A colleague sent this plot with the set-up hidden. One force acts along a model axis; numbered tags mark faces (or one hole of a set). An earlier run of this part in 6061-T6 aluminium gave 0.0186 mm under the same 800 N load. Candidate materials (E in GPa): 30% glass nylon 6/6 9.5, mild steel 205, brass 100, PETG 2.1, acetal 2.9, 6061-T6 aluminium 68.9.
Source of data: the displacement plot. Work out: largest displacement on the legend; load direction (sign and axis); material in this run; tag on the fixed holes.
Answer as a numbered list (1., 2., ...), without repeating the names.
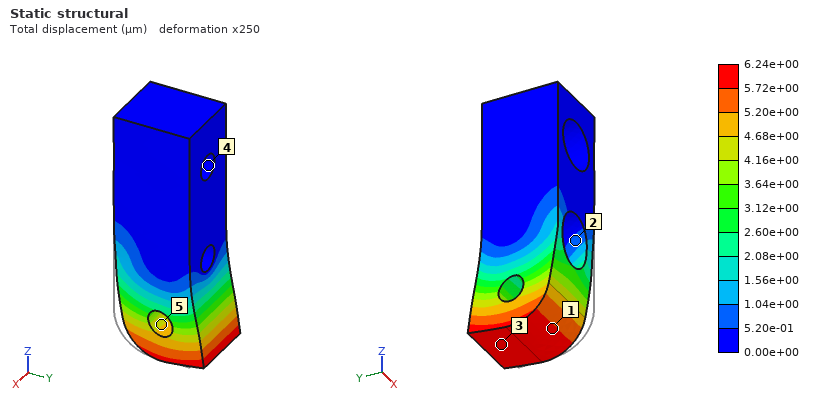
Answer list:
1. 6.24e+00 µm
2. +Y
3. mild steel
4. 4
